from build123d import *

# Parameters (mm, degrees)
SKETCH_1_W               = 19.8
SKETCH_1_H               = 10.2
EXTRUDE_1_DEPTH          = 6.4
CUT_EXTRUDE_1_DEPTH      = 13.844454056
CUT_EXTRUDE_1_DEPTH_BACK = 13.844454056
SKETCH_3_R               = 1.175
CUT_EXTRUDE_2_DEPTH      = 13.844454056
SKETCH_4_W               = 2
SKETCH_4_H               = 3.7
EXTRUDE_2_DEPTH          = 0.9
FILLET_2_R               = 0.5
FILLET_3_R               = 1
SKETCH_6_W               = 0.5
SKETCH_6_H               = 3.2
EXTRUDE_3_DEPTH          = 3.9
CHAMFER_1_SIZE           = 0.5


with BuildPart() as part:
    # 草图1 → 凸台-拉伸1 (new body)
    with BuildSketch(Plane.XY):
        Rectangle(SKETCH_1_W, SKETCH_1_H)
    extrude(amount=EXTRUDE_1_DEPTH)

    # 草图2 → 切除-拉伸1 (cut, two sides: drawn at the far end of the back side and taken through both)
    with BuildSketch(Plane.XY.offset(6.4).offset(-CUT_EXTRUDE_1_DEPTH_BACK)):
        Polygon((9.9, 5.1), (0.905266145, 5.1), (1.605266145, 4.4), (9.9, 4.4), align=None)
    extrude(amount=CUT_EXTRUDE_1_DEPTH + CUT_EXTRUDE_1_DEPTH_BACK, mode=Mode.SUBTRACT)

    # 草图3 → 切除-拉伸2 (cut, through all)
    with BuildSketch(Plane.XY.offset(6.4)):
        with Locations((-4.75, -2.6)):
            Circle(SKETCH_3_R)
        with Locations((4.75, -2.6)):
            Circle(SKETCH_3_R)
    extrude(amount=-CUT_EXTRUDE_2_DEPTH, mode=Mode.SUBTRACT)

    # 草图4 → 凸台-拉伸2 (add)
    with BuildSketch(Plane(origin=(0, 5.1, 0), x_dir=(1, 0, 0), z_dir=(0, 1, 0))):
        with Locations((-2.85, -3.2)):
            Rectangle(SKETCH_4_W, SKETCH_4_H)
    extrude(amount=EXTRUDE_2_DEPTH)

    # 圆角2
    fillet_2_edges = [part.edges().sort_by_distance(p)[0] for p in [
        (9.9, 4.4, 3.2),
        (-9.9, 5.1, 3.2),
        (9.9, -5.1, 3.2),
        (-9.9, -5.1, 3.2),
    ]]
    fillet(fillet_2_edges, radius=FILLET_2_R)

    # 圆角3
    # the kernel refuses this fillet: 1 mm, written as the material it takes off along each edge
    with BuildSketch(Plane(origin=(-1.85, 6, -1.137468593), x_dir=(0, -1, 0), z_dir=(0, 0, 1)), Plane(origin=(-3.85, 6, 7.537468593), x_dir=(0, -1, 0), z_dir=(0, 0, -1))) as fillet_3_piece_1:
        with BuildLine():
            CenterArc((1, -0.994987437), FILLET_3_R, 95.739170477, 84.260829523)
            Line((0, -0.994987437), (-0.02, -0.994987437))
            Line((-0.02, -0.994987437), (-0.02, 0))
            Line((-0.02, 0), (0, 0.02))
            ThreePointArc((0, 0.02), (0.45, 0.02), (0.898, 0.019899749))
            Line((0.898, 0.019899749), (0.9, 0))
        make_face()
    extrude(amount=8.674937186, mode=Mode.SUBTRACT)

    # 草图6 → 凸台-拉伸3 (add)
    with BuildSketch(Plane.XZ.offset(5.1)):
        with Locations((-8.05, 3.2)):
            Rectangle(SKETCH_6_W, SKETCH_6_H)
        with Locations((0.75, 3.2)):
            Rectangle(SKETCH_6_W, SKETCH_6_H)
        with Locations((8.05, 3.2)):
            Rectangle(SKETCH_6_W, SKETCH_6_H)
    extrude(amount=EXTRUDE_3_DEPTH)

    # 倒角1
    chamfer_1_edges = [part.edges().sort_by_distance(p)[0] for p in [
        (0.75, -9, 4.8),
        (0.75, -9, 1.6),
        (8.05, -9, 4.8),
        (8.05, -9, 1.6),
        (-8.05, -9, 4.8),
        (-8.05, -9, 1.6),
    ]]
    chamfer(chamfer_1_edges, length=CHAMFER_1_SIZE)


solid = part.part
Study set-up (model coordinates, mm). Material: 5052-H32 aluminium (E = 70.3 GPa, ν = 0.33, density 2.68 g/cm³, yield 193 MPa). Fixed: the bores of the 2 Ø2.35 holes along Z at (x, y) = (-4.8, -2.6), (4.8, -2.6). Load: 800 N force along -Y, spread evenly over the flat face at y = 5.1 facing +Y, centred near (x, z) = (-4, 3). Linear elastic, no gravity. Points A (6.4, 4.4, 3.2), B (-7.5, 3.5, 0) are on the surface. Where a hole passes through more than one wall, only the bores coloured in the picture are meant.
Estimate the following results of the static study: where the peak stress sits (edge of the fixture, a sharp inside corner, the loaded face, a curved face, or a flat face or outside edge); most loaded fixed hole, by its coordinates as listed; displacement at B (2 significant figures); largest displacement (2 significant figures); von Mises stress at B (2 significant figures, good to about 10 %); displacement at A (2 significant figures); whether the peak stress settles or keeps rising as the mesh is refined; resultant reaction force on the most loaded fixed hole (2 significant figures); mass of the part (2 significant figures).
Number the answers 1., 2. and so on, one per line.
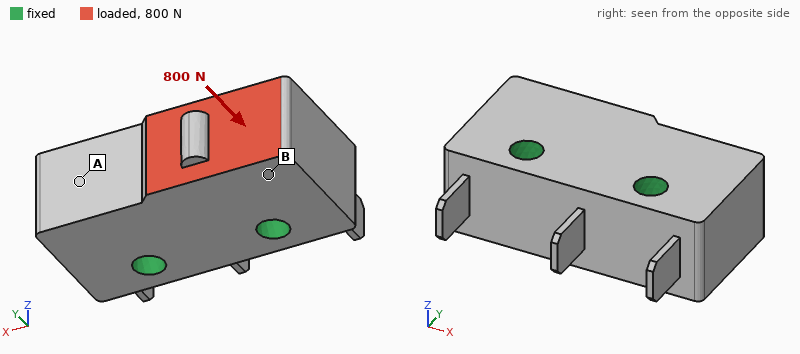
1. edge of the fixture
2. (-4.8, -2.6)
3. 2.0 µm
4. 2.5 µm
5. 15 MPa
6. 0.41 µm
7. keeps rising
8. 720 N
9. 3.3 g
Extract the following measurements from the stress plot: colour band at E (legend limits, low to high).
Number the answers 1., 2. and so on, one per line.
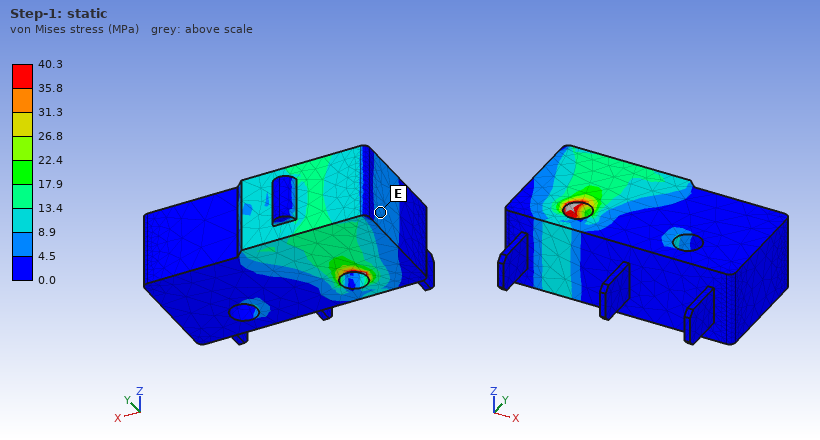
1. 4.5 to 8.9 MPa
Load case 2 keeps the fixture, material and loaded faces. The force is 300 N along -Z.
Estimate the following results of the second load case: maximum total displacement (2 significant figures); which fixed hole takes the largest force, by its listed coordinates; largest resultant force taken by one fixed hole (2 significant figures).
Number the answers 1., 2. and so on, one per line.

1. 5.0 µm
2. (-4.8, -2.6)
3. 240 N
